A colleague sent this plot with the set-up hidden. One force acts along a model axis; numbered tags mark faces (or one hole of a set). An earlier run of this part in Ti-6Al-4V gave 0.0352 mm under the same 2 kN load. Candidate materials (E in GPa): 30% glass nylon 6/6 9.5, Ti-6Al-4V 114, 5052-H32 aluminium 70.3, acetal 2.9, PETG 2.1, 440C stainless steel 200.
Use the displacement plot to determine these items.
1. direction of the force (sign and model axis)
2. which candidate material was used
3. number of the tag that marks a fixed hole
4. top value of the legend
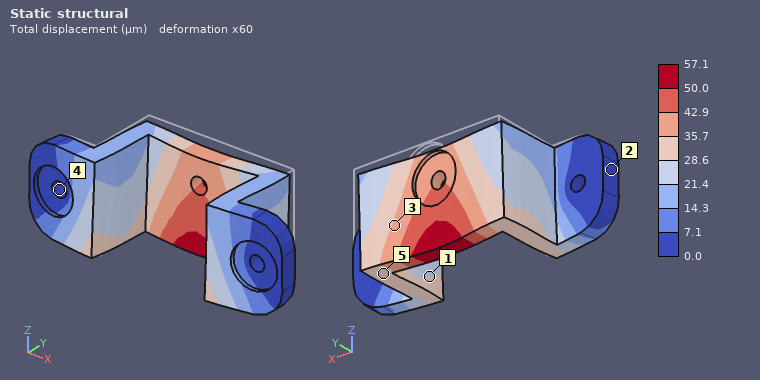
-Y
5052-H32 aluminium
4
57.1 µm
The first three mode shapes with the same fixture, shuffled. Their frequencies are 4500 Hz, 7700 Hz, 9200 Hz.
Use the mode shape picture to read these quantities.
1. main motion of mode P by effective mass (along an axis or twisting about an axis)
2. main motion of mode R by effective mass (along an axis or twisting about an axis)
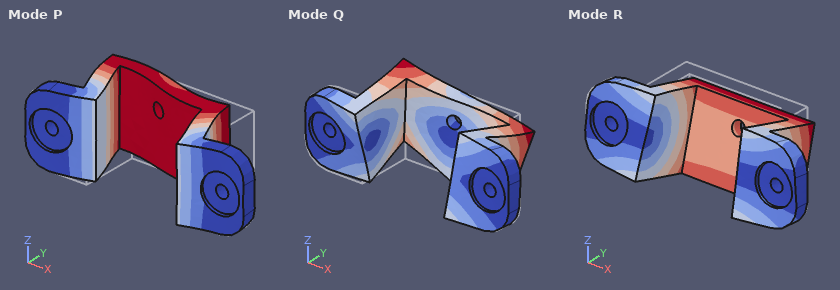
along X
along Z
